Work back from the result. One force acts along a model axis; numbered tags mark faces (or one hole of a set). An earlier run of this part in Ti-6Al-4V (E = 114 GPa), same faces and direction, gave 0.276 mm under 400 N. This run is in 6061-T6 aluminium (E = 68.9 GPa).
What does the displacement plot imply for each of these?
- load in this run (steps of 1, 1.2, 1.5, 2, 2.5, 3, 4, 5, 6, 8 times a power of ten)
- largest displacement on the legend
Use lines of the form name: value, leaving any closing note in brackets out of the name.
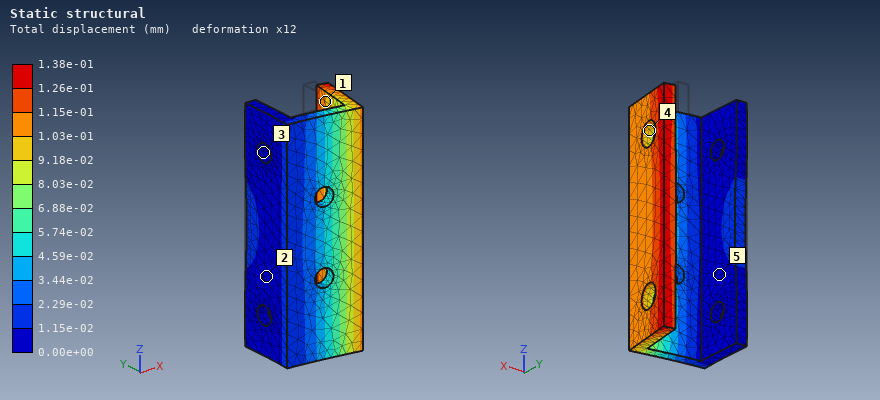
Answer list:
load in this run: 120 N
largest displacement on the legend: 1.38e-01 mm
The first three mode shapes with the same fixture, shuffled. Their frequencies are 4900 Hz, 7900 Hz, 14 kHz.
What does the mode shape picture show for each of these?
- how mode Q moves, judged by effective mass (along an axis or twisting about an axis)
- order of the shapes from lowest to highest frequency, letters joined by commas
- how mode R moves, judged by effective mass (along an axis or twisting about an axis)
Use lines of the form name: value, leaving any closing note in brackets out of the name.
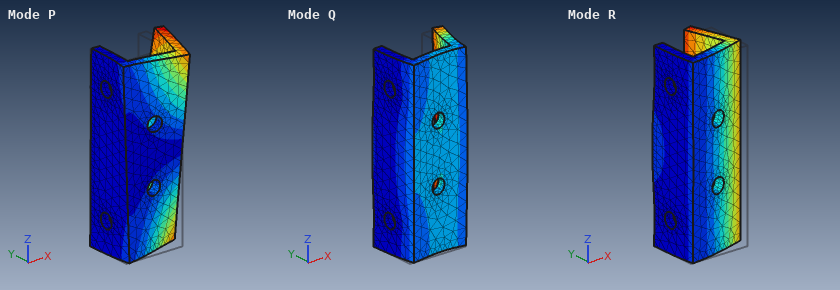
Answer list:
how mode Q moves, judged by effective mass: along X
order of the shapes from lowest to highest frequency, letters joined by commas: R, P, Q
how mode R moves, judged by effective mass: along Y
